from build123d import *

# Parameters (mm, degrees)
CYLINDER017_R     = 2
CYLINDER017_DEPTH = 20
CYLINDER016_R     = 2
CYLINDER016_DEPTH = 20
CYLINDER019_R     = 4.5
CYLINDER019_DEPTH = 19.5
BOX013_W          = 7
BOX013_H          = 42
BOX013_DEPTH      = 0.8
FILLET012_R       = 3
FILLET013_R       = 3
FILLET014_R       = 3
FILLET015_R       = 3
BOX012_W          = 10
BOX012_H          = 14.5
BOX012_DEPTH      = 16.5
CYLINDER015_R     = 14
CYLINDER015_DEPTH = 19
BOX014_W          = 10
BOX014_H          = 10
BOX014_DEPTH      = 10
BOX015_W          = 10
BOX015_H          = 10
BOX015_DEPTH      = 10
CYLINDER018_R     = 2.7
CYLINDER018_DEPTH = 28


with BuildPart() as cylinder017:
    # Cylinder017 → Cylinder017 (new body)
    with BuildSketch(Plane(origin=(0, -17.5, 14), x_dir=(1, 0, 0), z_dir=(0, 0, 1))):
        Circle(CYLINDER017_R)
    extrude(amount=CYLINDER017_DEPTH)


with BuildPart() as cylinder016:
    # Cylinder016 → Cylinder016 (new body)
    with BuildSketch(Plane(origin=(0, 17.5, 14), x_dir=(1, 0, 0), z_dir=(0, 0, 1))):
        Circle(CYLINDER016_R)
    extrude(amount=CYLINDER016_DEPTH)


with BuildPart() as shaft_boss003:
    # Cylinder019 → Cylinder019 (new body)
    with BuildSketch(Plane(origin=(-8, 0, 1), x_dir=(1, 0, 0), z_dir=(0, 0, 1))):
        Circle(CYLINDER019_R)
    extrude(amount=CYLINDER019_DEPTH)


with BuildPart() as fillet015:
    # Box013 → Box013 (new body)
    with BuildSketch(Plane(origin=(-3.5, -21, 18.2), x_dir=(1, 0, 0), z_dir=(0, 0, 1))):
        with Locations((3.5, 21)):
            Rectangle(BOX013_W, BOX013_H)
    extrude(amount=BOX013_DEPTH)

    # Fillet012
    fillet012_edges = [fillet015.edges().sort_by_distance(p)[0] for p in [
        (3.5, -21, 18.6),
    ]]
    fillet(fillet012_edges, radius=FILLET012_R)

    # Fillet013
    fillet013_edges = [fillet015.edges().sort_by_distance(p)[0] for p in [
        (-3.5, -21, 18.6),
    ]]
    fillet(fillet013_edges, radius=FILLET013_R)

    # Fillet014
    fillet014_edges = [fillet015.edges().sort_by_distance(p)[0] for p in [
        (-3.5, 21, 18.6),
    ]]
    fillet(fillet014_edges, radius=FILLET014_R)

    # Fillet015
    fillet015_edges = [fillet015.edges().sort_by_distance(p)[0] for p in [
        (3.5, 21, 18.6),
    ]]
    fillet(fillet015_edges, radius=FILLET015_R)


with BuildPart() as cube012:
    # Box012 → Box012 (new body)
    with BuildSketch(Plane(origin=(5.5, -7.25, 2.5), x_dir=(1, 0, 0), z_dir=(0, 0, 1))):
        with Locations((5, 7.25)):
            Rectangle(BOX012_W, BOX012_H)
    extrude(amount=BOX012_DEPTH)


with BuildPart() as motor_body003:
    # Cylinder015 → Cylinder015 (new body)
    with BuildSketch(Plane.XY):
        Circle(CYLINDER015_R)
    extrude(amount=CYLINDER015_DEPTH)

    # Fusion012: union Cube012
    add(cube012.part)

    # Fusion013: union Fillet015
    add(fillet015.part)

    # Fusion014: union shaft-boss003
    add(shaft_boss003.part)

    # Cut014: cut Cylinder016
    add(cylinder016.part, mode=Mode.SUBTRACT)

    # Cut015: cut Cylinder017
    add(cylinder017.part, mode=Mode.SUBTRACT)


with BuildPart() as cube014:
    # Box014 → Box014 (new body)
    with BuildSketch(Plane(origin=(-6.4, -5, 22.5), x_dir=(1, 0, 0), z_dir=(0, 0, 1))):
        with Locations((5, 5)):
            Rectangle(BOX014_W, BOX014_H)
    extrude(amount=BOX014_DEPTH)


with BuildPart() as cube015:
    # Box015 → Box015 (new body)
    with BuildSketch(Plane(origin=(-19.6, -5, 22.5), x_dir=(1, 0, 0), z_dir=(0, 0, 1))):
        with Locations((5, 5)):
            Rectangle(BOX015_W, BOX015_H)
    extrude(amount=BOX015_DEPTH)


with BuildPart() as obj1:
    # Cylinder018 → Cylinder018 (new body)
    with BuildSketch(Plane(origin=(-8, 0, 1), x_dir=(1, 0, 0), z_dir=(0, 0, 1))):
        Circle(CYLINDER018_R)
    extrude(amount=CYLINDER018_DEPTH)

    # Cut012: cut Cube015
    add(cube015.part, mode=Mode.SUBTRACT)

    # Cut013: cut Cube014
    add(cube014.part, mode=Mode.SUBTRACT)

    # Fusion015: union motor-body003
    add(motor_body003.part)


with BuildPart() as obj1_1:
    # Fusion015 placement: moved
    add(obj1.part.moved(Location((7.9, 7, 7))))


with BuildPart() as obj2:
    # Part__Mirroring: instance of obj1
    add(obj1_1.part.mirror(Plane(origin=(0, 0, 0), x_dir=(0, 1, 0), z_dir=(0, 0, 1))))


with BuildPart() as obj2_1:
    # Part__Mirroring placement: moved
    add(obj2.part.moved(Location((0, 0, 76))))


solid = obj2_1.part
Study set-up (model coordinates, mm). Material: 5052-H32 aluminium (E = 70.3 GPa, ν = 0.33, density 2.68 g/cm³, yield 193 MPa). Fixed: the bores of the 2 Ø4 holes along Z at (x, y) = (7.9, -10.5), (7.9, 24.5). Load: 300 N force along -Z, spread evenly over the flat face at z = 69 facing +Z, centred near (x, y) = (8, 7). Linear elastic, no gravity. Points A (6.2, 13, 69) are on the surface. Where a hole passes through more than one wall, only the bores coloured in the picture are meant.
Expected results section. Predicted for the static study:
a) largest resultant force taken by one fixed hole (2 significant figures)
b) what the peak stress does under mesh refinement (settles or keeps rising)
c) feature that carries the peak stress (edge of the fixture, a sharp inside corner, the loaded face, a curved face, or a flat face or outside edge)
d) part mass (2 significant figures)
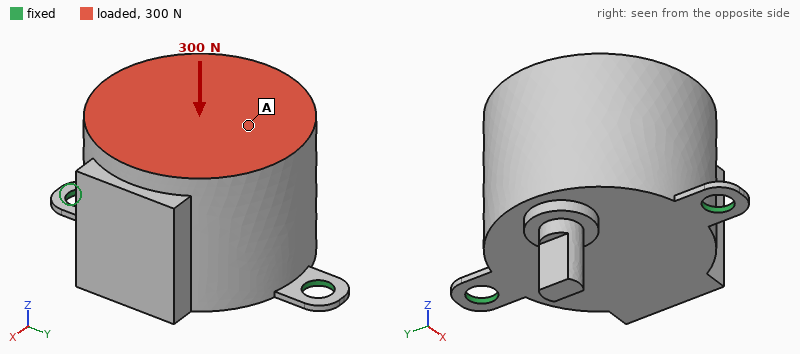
180 N
keeps rising
edge of the fixture
34 g
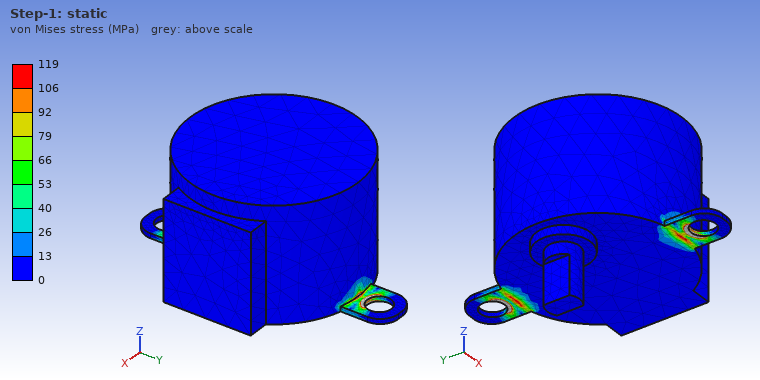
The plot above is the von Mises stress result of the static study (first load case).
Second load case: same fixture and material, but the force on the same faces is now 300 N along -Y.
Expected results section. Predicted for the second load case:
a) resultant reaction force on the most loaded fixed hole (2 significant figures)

240 N
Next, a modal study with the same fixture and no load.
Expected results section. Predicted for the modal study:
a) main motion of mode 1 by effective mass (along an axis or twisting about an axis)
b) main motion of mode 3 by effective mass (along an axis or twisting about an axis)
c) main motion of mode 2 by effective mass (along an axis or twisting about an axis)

along X
along Y
along Z
